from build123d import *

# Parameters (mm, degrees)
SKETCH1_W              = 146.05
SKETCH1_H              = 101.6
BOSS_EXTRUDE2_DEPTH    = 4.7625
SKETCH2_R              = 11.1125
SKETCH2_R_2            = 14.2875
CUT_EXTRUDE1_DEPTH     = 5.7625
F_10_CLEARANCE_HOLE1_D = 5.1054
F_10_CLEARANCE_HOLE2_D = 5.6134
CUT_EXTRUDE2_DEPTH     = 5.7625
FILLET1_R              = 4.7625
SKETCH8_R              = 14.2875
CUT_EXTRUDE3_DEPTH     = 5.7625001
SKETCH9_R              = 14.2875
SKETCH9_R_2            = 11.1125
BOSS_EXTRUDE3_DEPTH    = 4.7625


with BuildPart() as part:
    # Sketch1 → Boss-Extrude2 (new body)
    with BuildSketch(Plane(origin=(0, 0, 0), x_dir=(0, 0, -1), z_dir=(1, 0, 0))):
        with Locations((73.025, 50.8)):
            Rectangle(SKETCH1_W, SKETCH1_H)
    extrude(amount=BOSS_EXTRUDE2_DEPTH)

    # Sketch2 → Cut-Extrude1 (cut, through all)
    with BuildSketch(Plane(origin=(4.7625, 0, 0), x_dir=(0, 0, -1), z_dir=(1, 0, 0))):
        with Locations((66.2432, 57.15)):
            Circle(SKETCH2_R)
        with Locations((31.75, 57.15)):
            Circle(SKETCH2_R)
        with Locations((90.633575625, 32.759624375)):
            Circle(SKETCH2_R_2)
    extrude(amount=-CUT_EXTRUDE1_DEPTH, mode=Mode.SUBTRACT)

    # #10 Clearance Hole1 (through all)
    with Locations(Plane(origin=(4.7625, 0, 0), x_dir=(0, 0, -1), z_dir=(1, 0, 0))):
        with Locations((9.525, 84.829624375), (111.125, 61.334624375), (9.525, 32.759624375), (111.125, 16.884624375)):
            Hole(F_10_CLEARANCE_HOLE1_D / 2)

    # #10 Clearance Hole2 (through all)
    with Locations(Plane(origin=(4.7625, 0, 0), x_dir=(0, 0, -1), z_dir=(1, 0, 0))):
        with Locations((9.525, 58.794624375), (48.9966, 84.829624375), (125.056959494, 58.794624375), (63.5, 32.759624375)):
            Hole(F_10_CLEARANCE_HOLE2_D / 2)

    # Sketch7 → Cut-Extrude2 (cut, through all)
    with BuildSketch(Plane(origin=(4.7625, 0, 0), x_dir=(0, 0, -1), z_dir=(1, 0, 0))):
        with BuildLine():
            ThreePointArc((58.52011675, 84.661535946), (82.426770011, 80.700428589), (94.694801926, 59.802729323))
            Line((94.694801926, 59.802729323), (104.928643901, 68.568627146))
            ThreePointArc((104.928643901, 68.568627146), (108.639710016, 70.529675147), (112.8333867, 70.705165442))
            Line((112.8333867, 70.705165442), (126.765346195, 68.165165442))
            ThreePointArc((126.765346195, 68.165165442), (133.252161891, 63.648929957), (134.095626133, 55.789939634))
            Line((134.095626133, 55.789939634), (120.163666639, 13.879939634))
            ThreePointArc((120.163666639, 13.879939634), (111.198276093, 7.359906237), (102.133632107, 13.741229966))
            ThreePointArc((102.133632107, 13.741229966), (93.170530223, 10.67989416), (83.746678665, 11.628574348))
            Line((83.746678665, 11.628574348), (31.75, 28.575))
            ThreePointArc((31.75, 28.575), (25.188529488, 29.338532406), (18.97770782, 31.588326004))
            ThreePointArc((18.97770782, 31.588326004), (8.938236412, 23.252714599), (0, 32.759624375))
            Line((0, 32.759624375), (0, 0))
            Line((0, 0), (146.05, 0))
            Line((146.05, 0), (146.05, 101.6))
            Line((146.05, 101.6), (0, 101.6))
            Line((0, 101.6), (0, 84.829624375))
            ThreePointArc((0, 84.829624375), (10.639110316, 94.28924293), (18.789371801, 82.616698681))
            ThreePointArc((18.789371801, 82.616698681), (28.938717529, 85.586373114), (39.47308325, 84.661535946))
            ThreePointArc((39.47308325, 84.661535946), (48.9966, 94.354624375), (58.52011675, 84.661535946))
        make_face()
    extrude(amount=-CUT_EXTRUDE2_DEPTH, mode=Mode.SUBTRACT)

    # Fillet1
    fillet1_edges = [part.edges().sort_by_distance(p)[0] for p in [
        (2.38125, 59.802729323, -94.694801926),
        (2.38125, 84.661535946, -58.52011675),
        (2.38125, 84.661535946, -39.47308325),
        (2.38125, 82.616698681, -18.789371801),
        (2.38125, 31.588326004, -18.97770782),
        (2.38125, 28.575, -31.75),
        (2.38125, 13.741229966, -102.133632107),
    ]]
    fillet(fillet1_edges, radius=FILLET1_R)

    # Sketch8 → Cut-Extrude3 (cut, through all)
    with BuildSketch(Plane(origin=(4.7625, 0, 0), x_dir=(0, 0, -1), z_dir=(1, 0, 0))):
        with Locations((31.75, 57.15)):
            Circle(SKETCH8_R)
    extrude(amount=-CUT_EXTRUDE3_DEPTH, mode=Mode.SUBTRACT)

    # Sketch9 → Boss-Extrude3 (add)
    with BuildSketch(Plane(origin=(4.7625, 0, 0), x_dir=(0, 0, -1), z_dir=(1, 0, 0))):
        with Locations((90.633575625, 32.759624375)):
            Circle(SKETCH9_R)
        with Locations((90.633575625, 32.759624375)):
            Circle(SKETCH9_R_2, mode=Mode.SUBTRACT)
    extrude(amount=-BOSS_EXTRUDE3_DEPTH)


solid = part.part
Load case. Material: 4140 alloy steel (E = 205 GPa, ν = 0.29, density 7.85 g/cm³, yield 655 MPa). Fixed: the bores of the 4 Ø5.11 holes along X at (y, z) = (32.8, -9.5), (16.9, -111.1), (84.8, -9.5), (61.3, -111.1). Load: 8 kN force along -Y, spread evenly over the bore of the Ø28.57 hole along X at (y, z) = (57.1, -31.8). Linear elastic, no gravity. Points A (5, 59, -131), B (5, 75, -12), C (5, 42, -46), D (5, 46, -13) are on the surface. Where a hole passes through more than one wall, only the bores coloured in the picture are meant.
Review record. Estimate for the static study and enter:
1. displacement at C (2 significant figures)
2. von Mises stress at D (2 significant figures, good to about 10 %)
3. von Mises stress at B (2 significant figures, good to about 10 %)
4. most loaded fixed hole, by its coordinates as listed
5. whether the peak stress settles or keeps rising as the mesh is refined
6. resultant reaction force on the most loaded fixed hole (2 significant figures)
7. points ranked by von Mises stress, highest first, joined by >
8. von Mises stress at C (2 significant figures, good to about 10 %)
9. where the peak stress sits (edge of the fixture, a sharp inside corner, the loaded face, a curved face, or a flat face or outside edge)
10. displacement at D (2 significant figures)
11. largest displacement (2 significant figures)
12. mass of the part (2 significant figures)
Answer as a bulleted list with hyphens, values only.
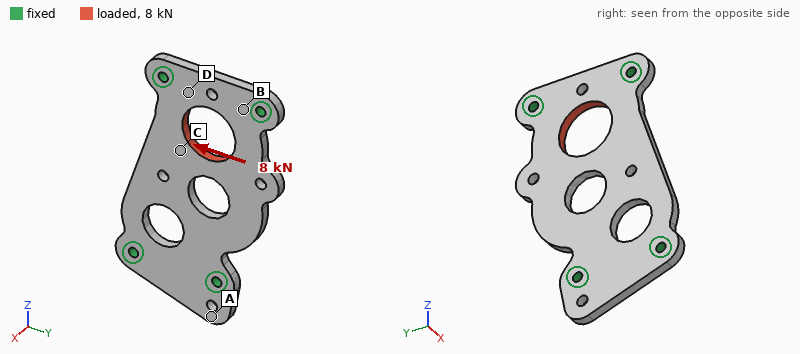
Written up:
- 16 µm
- 42 MPa
- 33 MPa
- (32.8, -9.5)
- keeps rising
- 3.5 kN
- D > B > C > A
- 16 MPa
- edge of the fixture
- 3.3 µm
- 17 µm
- 240 g
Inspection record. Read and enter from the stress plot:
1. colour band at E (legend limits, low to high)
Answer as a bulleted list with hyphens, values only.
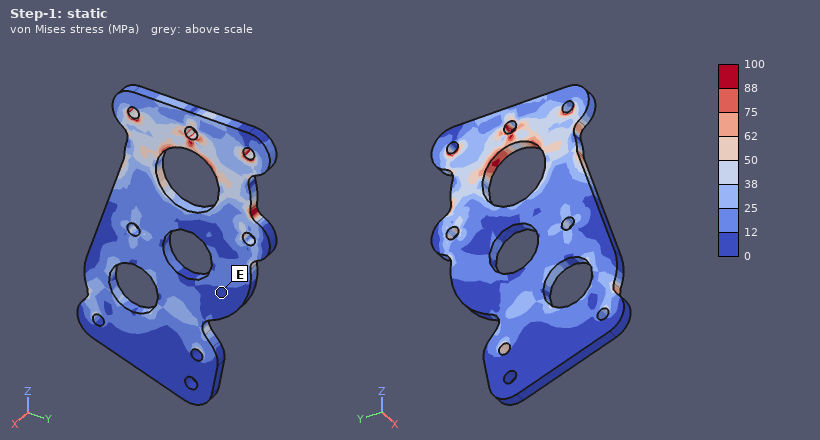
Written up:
- 0 to 12 MPa
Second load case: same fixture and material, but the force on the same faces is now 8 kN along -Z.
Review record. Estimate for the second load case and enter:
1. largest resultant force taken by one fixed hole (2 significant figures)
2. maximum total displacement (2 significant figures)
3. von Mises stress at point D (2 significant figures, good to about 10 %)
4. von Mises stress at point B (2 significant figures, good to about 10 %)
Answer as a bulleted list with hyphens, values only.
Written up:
- 3.2 kN
- 8.9 µm
- 27 MPa
- 28 MPa
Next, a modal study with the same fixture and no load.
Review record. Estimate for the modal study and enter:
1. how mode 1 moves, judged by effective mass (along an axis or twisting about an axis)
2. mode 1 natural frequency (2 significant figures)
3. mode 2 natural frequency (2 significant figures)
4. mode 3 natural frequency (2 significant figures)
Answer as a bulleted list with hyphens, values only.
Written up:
- along X
- 2100 Hz
- 2700 Hz
- 5600 Hz
